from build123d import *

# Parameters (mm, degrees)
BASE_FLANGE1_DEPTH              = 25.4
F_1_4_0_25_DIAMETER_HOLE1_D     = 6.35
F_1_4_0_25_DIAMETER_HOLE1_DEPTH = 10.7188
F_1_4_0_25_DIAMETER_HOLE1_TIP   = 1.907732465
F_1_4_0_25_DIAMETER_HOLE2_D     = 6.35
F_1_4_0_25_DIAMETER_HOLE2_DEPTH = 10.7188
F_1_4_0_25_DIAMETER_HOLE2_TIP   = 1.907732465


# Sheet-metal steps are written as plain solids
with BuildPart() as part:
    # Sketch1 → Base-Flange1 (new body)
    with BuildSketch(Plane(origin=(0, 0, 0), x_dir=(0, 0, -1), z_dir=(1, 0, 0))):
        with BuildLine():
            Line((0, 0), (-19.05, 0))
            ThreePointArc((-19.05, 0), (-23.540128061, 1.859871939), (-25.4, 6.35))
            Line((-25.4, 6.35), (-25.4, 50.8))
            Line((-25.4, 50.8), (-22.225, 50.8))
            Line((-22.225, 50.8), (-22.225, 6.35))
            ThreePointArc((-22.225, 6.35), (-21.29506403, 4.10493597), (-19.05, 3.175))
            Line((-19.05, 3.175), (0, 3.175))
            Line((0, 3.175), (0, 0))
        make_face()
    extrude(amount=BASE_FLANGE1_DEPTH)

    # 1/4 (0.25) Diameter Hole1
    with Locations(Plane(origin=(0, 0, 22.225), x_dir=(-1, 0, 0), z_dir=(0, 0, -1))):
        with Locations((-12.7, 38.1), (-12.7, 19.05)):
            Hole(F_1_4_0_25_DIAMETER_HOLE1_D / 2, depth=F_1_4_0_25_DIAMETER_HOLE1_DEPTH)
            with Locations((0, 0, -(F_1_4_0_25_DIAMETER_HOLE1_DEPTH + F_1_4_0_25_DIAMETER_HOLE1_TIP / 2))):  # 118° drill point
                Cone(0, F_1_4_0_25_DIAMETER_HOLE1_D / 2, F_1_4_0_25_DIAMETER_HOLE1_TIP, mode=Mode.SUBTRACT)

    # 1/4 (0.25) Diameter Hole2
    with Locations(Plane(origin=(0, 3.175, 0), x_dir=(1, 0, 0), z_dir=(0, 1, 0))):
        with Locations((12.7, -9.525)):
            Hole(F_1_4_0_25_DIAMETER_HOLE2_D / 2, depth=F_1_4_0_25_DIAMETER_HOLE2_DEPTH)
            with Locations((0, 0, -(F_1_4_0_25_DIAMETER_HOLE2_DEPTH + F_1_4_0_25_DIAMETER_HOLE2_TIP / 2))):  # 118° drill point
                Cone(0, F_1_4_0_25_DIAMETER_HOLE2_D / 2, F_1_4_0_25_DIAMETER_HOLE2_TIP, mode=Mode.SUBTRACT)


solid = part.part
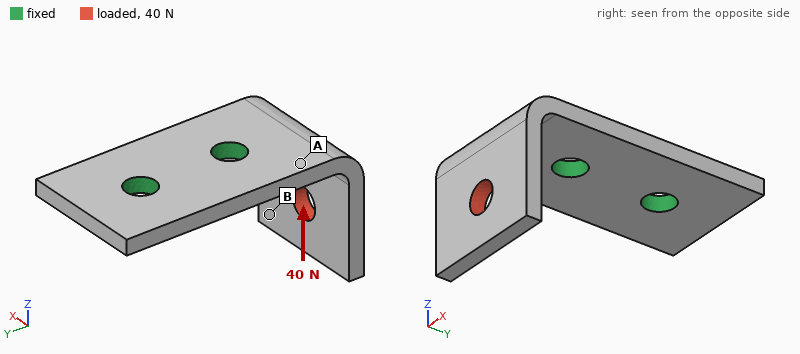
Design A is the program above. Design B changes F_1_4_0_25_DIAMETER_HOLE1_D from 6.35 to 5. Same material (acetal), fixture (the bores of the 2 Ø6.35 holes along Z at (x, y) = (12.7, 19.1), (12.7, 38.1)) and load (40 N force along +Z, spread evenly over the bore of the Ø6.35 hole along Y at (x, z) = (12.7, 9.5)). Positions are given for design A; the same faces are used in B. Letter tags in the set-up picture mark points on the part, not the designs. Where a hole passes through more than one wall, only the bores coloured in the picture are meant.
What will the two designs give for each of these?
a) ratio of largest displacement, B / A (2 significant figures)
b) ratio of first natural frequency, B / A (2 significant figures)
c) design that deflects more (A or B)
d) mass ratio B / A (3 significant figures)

1.1
0.96
B
1.01
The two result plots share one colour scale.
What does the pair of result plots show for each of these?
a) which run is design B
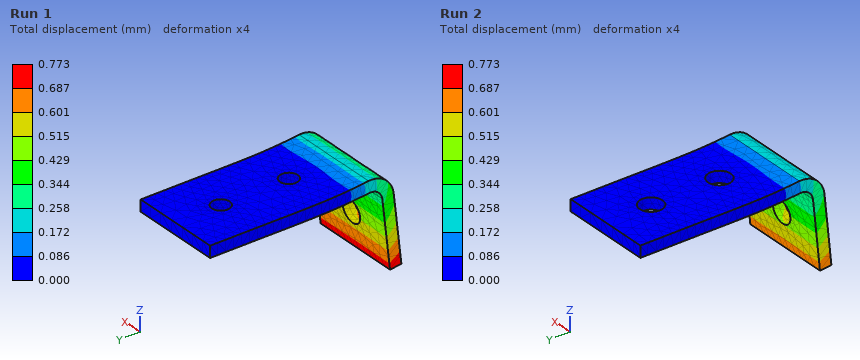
Run 1
